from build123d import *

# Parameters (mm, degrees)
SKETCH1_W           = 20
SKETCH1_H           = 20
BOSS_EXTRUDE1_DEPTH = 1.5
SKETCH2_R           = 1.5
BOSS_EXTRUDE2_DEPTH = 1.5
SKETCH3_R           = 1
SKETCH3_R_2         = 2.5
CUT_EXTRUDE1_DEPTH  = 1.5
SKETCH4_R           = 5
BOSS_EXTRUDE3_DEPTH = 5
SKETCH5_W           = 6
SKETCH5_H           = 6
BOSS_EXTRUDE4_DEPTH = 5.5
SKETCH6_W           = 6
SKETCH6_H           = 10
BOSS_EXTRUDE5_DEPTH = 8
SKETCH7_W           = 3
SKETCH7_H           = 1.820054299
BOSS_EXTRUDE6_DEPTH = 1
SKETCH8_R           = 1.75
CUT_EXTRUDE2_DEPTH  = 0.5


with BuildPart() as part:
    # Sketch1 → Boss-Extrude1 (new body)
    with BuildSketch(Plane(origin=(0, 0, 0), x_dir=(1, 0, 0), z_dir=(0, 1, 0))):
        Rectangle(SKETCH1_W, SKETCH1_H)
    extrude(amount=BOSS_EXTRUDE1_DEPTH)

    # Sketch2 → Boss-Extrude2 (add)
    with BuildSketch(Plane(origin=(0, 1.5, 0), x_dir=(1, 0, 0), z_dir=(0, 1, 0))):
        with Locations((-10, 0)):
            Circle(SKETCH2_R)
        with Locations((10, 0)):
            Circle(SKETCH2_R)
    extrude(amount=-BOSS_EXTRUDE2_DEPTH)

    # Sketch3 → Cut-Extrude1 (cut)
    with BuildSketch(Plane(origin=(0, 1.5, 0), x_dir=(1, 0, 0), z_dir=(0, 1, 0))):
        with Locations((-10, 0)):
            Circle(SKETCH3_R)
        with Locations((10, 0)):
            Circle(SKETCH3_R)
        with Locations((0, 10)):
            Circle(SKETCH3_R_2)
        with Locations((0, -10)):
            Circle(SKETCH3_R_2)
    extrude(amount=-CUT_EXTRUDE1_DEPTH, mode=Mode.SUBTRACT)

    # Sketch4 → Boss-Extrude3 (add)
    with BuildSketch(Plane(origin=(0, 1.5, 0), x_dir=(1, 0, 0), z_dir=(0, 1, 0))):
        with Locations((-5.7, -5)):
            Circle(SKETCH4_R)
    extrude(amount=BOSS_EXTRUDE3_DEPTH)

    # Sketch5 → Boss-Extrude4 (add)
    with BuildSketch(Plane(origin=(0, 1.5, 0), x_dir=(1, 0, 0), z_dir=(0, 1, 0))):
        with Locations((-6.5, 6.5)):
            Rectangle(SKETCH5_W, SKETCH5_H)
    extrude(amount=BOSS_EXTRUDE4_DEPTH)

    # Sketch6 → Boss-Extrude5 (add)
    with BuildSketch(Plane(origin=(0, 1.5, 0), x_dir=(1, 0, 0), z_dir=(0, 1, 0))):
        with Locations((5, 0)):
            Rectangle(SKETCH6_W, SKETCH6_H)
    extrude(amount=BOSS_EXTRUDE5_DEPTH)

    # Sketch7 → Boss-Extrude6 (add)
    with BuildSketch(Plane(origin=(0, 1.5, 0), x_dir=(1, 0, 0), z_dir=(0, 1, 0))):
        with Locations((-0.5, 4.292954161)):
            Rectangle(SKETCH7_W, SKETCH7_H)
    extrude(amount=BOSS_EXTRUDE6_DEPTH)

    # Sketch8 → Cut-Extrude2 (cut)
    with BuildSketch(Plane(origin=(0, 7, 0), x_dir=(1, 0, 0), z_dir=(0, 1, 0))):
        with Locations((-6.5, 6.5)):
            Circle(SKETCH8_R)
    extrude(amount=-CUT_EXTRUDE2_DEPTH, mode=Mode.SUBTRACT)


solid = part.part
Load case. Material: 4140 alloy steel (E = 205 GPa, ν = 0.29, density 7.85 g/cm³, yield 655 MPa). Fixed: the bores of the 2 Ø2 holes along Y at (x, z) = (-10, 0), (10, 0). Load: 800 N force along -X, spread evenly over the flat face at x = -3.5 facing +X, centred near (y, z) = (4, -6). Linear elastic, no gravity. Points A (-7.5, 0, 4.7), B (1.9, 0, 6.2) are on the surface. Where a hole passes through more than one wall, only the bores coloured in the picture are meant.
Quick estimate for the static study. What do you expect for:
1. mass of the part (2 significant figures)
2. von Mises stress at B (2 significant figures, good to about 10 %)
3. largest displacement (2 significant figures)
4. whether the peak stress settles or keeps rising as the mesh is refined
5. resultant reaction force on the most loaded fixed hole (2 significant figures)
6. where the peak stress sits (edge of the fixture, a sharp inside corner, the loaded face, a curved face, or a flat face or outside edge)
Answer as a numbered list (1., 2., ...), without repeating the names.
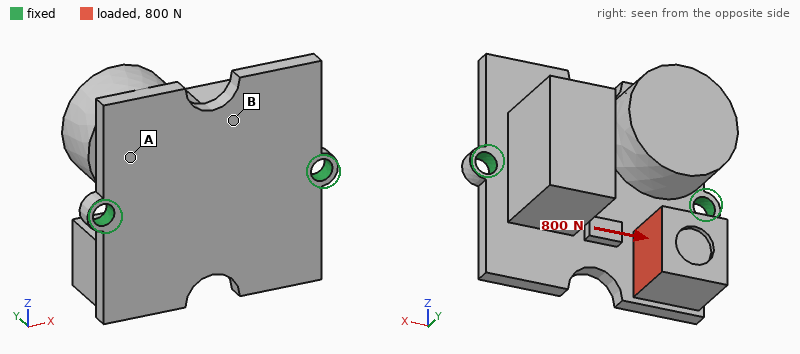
1. 13 g
2. 94 MPa
3. 53 µm
4. keeps rising
5. 510 N
6. edge of the fixture
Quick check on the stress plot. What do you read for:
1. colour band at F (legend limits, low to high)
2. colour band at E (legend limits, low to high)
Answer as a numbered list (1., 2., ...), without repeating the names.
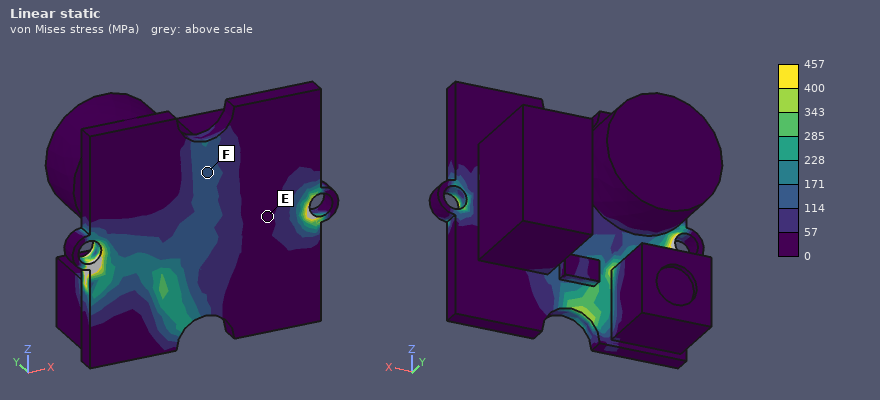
1. 114 to 171 MPa
2. 0 to 57 MPa
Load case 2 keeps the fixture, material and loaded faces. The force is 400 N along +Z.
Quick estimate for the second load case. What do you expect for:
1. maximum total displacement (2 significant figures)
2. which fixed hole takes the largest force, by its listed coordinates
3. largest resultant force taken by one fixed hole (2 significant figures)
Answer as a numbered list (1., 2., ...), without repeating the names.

1. 77 µm
2. (-10, 0)
3. 270 N
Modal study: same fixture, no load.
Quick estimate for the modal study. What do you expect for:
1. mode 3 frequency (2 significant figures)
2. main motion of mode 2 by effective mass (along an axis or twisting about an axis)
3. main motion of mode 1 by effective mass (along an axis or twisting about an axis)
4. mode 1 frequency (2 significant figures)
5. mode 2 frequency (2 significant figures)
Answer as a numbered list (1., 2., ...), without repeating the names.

1. 11 kHz
2. along Y
3. along Z
4. 5600 Hz
5. 7800 Hz
